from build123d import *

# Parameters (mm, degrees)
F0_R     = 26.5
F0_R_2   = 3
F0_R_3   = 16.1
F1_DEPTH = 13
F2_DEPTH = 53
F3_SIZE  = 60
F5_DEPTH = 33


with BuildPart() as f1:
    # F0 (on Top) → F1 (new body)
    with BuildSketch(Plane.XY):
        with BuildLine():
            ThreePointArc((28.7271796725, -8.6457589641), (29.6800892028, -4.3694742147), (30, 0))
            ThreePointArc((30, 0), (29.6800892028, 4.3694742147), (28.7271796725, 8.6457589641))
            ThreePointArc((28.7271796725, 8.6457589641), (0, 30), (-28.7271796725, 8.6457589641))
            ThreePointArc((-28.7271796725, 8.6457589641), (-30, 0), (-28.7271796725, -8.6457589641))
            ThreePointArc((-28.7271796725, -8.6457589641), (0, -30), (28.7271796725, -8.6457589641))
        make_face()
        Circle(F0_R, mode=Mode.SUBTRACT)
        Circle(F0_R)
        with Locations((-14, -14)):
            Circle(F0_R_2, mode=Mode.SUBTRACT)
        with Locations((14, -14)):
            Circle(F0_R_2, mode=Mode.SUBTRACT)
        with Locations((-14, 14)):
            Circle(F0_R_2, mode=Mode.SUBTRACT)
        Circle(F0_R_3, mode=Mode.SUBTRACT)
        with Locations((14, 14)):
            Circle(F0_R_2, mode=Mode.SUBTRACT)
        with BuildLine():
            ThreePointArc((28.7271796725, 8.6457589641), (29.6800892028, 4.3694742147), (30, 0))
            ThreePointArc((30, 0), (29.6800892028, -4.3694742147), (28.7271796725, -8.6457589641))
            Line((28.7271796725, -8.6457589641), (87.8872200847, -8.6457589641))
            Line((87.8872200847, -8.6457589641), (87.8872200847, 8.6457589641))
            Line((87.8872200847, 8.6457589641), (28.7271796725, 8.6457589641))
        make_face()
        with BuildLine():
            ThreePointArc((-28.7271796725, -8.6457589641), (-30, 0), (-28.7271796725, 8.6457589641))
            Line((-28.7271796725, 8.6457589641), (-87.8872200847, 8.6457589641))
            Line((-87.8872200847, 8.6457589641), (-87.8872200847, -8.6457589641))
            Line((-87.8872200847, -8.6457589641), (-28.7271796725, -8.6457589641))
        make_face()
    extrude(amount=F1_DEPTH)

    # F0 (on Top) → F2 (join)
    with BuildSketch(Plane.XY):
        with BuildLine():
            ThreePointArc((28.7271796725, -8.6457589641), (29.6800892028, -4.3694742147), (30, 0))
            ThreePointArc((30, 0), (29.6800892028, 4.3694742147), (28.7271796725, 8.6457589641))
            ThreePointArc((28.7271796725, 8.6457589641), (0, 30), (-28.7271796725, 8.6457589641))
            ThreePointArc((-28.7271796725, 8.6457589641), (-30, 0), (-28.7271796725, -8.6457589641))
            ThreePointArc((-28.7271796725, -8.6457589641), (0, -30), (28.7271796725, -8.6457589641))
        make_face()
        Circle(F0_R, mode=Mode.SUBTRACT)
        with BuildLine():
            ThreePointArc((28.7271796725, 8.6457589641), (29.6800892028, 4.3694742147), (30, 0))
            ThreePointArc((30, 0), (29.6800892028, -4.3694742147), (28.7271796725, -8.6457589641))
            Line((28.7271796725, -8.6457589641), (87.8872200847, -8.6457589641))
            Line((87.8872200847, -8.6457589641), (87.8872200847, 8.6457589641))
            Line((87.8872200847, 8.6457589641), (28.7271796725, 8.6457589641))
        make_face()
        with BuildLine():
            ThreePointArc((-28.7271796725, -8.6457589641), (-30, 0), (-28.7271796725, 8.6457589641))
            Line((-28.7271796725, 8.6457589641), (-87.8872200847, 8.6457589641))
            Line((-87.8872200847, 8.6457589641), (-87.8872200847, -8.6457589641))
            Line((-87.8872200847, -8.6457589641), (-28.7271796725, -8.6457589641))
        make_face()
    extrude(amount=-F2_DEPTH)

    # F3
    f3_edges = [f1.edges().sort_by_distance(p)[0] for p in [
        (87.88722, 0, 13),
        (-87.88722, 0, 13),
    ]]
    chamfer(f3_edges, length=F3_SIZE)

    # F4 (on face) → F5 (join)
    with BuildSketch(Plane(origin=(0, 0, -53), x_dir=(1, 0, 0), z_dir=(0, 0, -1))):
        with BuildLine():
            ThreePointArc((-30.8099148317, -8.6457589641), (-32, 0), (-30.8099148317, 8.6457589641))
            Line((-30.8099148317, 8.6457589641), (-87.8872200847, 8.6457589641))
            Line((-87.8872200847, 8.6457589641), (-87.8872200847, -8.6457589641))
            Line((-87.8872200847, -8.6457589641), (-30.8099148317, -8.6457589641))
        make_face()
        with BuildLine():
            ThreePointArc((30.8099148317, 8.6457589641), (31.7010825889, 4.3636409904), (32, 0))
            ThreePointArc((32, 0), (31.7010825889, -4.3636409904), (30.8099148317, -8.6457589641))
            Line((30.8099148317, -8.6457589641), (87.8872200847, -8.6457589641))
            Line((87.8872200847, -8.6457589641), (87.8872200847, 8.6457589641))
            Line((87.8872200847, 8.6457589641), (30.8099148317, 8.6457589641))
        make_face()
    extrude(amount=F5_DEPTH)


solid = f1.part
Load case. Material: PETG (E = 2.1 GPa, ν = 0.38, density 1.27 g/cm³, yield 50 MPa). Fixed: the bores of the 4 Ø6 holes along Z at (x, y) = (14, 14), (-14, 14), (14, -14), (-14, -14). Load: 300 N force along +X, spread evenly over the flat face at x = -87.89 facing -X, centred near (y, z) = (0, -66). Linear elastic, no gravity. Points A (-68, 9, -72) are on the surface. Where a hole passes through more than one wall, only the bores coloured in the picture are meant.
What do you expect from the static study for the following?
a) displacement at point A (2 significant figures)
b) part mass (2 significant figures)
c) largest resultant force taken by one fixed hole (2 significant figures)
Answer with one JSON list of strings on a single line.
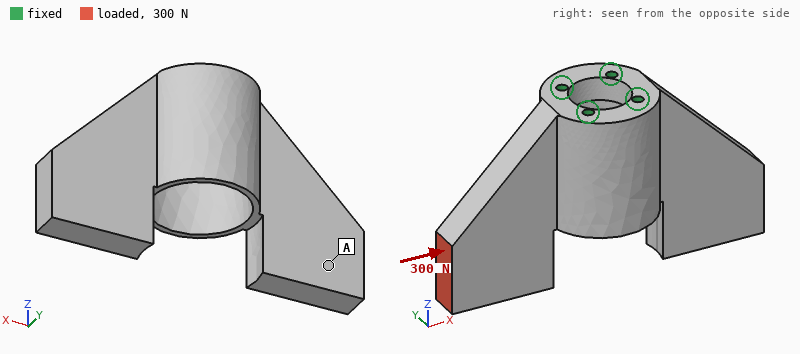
["1.2 mm", "240 g", "250 N"]
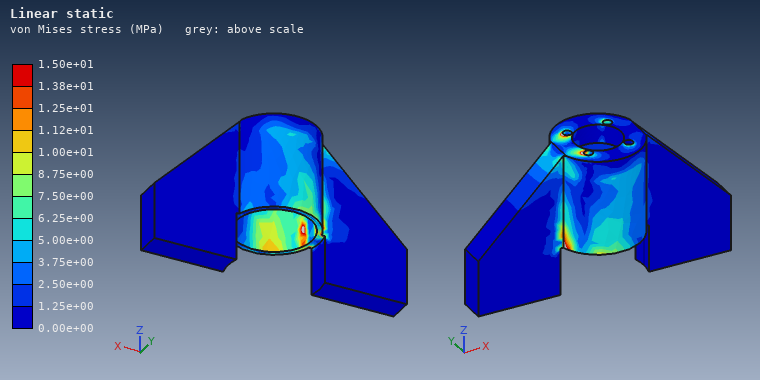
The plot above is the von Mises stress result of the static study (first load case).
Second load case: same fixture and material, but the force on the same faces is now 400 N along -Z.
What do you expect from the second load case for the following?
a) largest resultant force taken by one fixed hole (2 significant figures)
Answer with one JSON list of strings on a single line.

["500 N"]
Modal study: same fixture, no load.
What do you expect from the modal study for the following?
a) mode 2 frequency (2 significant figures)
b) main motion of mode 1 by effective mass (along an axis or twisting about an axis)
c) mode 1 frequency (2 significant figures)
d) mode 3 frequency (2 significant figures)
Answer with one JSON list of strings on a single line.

["350 Hz", "along Z", "270 Hz", "350 Hz"]
